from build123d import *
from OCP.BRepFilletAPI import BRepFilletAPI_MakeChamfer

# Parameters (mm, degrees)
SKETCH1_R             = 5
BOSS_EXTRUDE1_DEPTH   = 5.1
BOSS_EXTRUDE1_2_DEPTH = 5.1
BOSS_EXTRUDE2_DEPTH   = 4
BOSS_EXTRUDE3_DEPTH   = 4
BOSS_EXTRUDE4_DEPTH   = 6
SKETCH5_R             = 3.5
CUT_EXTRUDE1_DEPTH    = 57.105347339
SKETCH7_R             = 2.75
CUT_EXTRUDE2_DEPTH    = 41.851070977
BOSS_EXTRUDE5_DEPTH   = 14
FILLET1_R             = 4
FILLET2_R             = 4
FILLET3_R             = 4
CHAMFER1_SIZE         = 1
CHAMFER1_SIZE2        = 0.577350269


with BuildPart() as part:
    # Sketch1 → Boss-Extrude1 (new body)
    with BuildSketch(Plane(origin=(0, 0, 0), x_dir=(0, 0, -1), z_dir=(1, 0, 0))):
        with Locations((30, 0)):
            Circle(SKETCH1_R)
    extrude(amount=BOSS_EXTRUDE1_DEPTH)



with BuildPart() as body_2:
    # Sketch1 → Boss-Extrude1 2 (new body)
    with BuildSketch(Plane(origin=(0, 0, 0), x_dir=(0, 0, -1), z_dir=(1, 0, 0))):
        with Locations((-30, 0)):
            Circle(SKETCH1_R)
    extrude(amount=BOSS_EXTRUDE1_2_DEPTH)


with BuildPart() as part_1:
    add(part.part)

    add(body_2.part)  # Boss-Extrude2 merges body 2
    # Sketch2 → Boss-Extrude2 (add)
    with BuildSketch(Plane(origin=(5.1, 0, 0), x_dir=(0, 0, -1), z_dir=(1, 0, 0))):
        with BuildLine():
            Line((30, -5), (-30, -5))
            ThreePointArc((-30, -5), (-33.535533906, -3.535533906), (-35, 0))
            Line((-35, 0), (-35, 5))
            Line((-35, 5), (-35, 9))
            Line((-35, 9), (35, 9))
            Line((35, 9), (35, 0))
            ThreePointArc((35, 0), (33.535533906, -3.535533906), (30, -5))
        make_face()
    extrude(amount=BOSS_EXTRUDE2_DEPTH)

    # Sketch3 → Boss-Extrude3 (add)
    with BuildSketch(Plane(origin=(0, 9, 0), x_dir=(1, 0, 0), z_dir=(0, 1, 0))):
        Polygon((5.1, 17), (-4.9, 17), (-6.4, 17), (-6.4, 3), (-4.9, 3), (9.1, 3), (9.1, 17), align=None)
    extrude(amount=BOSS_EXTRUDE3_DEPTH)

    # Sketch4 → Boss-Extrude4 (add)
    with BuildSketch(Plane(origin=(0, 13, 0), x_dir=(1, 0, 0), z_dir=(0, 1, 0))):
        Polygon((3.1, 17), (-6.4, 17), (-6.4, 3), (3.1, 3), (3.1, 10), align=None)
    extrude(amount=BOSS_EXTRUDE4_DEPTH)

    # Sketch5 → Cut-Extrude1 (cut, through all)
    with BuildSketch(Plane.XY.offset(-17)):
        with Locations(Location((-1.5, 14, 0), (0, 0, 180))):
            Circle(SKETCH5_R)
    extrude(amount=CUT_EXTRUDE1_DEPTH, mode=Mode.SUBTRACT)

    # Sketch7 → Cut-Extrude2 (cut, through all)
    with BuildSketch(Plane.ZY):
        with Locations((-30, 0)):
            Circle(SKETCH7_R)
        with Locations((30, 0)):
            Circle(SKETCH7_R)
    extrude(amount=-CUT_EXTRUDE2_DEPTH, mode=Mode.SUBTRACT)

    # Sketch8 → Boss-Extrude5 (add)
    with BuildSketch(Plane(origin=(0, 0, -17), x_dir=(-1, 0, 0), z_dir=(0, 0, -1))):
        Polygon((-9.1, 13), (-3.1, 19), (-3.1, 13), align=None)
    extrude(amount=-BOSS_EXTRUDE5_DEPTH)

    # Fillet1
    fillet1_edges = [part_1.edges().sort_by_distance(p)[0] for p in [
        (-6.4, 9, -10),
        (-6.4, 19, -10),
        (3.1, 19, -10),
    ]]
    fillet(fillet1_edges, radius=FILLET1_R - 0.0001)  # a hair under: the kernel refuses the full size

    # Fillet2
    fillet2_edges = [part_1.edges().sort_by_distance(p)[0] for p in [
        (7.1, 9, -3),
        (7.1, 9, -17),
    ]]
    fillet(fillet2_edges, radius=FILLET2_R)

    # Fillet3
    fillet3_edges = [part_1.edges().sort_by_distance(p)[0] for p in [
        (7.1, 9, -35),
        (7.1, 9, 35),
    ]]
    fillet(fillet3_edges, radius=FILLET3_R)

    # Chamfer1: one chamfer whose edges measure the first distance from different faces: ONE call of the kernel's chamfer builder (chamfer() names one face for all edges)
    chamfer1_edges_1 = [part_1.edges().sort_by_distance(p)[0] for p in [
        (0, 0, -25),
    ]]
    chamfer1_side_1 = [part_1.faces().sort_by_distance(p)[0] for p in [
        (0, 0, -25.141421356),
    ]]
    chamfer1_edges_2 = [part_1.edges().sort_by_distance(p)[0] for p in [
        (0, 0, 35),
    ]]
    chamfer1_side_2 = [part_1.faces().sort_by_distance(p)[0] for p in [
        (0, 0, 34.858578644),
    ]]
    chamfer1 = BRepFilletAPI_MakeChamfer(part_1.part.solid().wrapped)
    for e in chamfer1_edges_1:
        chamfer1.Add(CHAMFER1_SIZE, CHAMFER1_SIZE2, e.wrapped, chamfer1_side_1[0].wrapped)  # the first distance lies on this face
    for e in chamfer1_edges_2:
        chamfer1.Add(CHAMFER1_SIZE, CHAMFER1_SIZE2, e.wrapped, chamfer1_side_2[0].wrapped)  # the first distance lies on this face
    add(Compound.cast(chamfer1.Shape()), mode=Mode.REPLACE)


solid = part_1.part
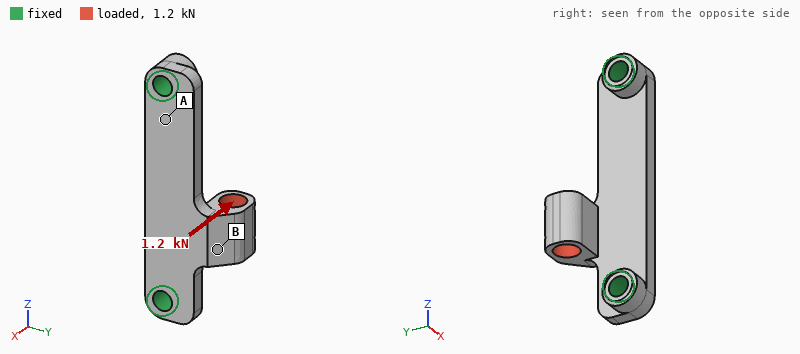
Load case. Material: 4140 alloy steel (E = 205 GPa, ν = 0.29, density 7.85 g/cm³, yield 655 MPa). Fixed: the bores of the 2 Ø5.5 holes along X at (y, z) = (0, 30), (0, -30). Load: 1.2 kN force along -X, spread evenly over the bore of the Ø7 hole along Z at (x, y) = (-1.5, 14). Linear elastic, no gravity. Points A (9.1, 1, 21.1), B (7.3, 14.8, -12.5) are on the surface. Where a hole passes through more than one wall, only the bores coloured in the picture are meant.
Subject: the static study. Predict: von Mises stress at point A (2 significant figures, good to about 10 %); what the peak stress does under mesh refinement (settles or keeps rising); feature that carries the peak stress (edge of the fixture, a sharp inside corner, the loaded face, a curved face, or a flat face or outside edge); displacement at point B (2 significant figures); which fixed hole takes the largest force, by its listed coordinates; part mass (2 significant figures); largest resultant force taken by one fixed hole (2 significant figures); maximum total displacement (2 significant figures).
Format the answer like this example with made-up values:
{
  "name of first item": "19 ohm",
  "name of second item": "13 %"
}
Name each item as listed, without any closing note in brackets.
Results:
{
  "von Mises stress at point A": "130 MPa",
  "what the peak stress does under mesh refinement": "keeps rising",
  "feature that carries the peak stress": "edge of the fixture",
  "displacement at point B": "0.13 mm",
  "which fixed hole takes the largest force, by its listed coordinates": "(0, -30)",
  "part mass": "43 g",
  "largest resultant force taken by one fixed hole": "880 N",
  "maximum total displacement": "0.21 mm"
}
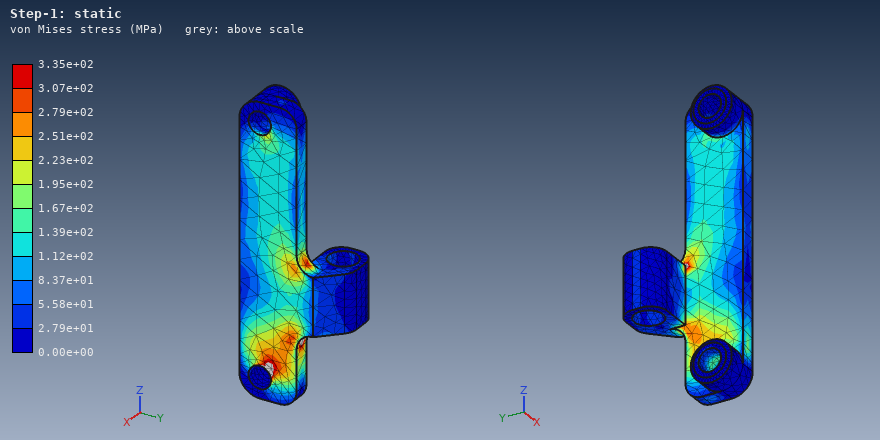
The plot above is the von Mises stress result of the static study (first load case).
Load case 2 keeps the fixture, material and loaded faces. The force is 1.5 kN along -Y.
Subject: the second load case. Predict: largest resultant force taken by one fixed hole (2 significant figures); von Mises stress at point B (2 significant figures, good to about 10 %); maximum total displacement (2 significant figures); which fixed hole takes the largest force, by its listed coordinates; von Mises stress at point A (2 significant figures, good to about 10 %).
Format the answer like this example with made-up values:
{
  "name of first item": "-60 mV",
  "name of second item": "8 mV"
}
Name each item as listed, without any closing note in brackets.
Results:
{
  "largest resultant force taken by one fixed hole": "1.1 kN",
  "von Mises stress at point B": "79 MPa",
  "maximum total displacement": "0.19 mm",
  "which fixed hole takes the largest force, by its listed coordinates": "(0, -30)",
  "von Mises stress at point A": "78 MPa"
}
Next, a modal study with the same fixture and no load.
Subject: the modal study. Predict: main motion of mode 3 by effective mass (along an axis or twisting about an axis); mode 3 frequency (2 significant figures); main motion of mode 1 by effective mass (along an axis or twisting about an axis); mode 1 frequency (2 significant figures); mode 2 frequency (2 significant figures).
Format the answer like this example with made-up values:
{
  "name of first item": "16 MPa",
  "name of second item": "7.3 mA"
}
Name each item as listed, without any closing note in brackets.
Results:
{
  "main motion of mode 3 by effective mass": "along Y",
  "mode 3 frequency": "12 kHz",
  "main motion of mode 1 by effective mass": "along X",
  "mode 1 frequency": "4100 Hz",
  "mode 2 frequency": "6800 Hz"
}
